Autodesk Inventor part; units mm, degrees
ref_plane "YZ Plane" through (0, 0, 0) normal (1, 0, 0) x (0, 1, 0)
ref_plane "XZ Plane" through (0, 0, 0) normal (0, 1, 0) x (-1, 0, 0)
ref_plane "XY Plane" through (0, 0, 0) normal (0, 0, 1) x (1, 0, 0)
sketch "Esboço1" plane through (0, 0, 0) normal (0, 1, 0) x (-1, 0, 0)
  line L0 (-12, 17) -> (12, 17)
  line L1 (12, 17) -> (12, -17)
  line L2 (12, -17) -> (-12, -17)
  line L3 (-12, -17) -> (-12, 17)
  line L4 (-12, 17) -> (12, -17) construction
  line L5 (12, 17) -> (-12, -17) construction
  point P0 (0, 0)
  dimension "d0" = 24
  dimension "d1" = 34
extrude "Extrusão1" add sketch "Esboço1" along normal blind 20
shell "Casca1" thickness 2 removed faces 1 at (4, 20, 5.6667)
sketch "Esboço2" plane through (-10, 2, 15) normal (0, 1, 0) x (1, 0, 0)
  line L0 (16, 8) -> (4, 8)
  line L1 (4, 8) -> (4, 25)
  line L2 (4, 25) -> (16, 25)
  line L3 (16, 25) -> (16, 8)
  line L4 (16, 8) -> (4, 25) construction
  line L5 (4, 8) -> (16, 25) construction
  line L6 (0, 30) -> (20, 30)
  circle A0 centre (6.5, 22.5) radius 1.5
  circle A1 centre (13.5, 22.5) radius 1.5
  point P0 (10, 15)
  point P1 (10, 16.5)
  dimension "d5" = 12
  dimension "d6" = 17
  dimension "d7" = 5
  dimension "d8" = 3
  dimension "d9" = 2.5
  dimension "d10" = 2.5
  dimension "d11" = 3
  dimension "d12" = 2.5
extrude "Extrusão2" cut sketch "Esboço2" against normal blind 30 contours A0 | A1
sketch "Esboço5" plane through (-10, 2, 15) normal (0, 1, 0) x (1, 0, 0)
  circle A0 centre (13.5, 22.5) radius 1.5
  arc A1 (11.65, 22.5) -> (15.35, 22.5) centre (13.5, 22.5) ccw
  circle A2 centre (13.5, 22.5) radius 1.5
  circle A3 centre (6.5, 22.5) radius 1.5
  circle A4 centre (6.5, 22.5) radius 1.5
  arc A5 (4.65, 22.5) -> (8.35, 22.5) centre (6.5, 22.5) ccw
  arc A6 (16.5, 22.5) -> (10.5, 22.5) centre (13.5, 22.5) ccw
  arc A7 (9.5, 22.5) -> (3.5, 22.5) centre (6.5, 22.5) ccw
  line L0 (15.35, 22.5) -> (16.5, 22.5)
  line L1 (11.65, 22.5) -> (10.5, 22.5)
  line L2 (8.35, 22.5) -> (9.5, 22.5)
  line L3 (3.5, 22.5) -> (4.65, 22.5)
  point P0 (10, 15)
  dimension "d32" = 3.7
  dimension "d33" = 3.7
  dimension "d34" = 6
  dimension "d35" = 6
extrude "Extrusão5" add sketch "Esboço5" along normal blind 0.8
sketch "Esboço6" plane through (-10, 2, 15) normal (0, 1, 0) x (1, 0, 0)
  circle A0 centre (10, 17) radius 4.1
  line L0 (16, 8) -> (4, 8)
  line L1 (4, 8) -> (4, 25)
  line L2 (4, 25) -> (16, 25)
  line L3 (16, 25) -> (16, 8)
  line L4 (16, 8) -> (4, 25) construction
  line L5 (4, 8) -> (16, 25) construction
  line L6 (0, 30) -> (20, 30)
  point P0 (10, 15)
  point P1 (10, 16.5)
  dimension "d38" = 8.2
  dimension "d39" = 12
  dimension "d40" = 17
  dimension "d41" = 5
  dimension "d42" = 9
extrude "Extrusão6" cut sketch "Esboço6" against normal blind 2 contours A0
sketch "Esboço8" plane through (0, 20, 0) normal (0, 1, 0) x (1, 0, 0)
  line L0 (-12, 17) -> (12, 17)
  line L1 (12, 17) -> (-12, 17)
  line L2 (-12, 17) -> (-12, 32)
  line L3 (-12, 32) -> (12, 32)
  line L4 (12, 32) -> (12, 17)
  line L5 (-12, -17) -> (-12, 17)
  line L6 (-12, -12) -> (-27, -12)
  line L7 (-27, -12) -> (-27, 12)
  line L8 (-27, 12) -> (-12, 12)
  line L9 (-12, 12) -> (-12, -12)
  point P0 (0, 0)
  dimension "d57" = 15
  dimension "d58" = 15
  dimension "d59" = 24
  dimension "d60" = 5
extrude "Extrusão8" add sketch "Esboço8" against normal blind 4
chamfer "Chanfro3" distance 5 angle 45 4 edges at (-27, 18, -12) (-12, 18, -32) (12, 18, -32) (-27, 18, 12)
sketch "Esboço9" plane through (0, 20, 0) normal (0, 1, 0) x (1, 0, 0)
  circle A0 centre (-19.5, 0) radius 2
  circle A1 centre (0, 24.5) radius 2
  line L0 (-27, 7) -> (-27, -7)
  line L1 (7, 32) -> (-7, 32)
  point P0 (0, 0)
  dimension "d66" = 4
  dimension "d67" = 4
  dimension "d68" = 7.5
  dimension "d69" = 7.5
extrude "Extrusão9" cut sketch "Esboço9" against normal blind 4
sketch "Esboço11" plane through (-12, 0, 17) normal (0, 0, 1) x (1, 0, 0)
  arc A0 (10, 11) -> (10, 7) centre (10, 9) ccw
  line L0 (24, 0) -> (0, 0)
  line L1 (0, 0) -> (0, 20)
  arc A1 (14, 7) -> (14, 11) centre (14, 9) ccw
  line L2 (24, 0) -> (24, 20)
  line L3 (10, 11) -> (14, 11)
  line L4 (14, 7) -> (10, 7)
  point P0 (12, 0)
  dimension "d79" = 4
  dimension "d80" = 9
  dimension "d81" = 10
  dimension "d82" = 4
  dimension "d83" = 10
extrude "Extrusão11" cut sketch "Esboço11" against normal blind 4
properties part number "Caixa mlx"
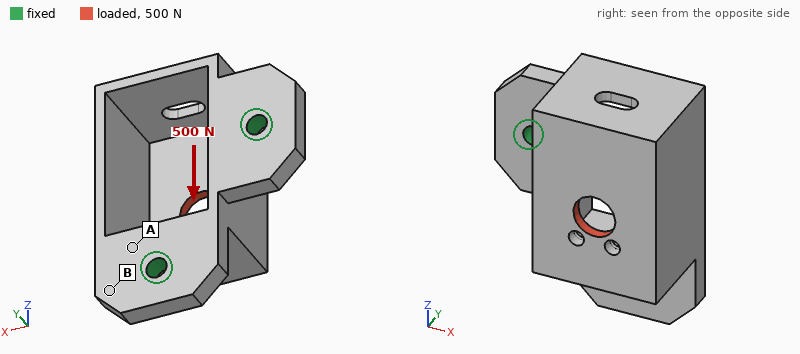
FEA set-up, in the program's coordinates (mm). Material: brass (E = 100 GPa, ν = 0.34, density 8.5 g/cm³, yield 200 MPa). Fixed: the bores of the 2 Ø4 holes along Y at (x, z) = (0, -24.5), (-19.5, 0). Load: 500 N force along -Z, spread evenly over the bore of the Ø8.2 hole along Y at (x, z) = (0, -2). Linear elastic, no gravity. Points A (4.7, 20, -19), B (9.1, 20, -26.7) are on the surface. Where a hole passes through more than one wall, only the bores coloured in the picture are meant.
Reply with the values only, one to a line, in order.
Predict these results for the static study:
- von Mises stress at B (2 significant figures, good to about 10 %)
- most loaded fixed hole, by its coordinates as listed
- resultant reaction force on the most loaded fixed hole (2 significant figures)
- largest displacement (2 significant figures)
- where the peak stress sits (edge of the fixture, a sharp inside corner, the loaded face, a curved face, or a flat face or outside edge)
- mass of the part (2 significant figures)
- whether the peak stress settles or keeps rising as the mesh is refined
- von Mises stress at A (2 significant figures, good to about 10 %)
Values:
11 MPa
(0, -24.5)
430 N
75 µm
edge of the fixture
67 g
keeps rising
21 MPa
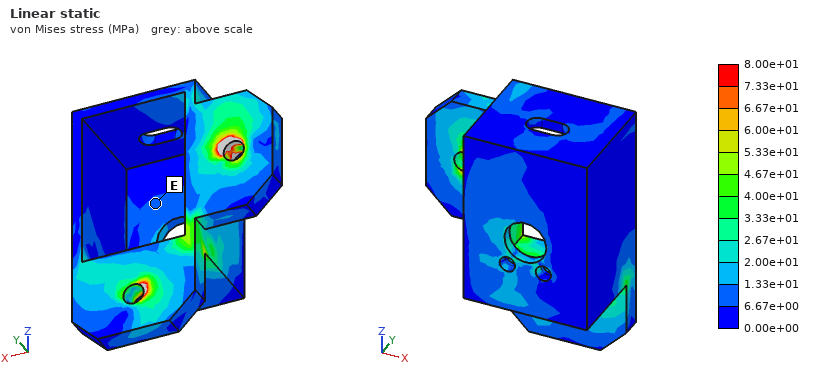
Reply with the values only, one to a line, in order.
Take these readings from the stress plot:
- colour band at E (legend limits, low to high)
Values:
6.67e+00 to 1.33e+01 MPa
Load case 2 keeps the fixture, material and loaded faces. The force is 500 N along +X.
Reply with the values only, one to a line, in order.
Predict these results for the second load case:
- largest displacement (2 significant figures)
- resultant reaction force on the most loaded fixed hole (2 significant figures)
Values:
95 µm
360 N
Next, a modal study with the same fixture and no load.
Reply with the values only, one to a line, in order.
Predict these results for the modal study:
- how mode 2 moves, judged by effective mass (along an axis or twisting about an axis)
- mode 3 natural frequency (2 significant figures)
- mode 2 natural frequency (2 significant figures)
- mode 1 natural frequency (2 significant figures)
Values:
along X
6200 Hz
4400 Hz
2000 Hz
